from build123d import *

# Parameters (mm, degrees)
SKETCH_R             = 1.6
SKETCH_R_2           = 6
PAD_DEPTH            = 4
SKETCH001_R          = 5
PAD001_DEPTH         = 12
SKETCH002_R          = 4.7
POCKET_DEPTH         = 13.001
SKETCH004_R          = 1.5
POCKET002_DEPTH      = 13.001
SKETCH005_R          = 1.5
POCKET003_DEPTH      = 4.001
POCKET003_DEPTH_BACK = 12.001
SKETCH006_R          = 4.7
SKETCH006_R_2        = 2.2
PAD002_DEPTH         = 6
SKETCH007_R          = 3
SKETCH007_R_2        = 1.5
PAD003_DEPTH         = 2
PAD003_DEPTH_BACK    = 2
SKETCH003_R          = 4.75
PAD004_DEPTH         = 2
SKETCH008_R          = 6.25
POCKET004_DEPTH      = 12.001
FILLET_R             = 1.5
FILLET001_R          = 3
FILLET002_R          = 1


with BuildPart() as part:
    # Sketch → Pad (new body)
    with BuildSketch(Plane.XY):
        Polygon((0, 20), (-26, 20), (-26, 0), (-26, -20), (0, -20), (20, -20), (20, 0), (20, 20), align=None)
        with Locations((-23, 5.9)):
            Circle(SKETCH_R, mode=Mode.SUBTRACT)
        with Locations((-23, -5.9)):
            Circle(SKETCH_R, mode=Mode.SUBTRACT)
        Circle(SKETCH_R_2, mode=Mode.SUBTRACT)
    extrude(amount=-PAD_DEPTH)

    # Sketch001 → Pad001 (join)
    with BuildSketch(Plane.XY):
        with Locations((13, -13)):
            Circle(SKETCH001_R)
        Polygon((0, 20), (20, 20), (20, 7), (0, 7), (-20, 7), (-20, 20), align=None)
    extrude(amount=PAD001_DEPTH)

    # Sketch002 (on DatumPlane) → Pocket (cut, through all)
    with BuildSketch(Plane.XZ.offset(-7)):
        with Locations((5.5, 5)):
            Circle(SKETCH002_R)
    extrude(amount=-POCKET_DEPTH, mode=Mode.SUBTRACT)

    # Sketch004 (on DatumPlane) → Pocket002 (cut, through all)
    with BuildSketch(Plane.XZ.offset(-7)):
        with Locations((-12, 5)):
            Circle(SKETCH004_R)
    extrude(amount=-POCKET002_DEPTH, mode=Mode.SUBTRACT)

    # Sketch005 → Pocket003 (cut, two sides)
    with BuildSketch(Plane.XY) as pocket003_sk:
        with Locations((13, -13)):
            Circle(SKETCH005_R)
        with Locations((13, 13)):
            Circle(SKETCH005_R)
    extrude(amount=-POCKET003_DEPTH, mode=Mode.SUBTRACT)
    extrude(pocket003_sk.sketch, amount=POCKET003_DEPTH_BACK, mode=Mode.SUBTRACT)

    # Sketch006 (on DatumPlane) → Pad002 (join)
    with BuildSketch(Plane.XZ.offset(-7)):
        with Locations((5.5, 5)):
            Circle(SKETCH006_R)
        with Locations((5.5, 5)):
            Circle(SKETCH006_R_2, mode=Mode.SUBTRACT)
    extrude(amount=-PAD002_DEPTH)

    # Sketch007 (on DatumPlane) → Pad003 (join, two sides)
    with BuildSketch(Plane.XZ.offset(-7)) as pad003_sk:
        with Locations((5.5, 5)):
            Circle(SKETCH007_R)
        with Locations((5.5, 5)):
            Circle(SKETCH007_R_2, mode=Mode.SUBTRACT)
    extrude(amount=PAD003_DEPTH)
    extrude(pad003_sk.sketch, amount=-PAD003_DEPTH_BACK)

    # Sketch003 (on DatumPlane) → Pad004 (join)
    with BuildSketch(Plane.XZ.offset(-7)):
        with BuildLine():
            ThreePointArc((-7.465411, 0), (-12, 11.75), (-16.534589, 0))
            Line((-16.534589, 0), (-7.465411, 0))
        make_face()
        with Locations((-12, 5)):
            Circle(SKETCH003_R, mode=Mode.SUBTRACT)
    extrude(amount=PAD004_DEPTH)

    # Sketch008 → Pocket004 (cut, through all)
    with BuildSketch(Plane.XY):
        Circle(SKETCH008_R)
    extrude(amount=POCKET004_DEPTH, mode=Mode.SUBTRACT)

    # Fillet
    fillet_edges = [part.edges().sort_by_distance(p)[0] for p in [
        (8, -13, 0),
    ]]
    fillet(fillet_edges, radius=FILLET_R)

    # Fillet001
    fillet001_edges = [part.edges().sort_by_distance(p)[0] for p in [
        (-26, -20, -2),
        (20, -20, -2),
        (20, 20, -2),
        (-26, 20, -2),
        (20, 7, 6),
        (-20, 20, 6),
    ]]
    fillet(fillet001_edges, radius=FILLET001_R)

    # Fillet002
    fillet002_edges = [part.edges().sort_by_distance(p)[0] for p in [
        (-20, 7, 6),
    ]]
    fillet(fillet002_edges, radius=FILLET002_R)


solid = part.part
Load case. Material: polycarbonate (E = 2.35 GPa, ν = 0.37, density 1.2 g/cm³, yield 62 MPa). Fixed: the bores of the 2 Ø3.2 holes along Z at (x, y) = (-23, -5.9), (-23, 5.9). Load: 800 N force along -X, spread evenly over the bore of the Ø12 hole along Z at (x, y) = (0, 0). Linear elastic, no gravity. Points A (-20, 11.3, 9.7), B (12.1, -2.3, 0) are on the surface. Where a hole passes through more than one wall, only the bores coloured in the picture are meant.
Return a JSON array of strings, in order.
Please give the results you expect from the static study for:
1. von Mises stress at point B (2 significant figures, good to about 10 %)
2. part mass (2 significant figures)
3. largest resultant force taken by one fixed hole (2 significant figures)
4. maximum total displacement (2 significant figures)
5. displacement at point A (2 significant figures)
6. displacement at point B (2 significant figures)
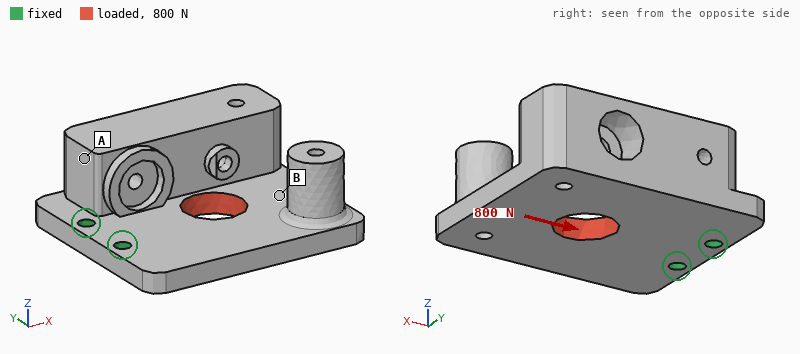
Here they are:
["3.1 MPa", "16 g", "400 N", "0.15 mm", "0.034 mm", "0.12 mm"]
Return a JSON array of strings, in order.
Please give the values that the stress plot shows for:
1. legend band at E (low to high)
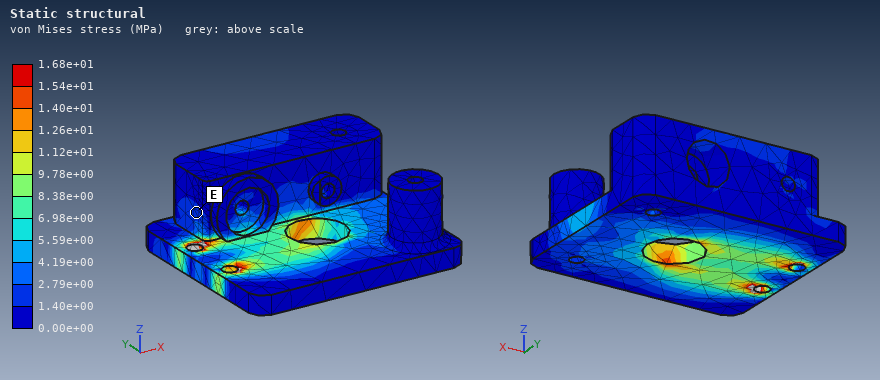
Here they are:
["1.40e+00 to 2.79e+00 MPa"]
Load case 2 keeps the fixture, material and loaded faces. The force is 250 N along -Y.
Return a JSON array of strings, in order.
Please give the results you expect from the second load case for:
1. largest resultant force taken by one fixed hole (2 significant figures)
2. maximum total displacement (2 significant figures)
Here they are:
["400 N", "0.40 mm"]
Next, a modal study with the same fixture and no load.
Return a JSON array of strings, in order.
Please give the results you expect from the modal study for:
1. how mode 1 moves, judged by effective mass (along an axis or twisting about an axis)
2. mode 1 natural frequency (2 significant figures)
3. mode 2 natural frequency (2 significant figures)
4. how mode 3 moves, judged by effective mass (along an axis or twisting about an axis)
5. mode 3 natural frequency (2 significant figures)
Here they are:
["along Z", "360 Hz", "770 Hz", "along Y", "1200 Hz"]
